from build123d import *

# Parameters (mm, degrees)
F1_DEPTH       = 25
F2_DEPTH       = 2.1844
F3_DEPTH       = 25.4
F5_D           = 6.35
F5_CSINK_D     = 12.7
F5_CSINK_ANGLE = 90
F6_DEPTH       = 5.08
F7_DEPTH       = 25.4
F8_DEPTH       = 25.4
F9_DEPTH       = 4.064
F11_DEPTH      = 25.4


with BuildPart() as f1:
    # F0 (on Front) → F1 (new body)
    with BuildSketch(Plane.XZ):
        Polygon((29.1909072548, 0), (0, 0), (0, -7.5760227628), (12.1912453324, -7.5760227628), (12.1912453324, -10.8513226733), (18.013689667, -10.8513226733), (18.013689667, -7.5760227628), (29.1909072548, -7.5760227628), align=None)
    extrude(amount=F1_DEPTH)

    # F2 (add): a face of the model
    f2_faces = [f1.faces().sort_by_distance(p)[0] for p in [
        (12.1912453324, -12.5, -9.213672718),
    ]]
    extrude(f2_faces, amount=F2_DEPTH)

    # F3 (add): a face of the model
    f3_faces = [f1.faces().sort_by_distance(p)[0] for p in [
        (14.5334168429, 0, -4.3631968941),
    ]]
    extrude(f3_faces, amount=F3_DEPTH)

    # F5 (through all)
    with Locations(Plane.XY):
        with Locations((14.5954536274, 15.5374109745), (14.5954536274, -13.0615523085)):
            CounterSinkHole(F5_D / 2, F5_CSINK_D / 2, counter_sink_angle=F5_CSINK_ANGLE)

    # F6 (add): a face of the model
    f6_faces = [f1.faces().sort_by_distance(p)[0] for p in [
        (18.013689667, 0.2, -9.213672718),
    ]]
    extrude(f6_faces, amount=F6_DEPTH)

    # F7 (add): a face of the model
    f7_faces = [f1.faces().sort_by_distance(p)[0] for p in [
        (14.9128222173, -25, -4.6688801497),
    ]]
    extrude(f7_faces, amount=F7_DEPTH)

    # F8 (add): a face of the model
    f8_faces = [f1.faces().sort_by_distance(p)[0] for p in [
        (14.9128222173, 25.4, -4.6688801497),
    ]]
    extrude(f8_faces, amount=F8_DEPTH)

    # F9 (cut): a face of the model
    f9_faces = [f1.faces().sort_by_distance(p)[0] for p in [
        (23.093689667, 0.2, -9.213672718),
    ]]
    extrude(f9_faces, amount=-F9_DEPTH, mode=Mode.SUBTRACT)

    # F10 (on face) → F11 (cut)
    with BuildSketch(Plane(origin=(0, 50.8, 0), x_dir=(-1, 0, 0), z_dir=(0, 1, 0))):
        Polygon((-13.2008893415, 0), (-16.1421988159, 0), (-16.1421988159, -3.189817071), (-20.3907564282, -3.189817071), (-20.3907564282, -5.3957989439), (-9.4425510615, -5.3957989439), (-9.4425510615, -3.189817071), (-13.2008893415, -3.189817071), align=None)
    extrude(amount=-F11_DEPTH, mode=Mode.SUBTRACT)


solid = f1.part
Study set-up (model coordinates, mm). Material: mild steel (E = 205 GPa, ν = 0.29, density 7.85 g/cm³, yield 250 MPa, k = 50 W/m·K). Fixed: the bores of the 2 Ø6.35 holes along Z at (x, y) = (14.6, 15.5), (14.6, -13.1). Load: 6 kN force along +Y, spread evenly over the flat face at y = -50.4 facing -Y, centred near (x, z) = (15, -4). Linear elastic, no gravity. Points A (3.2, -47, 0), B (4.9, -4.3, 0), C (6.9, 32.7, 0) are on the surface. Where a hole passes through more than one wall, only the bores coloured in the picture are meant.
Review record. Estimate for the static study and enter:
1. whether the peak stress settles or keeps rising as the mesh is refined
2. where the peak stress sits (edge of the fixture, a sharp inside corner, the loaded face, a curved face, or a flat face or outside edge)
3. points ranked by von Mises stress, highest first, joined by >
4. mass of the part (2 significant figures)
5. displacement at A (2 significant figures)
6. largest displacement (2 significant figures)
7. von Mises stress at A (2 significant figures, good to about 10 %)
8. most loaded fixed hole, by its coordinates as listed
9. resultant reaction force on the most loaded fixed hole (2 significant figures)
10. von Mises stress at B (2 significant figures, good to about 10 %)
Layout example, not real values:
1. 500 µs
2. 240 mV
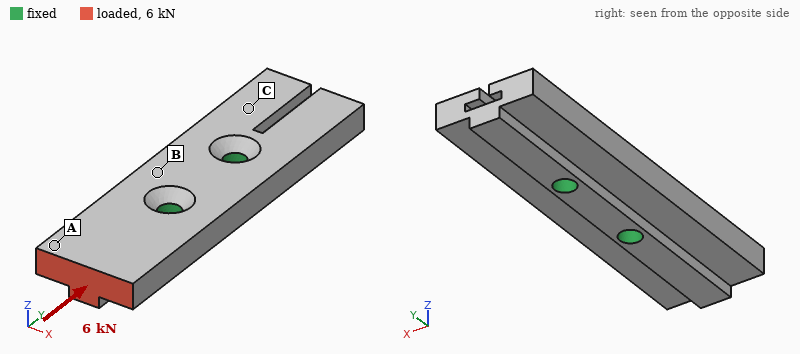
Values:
1. keeps rising
2. edge of the fixture
3. A > B > C
4. 180 g
5. 8.1 µm
6. 8.8 µm
7. 24 MPa
8. (14.6, -13.1)
9. 4.9 kN
10. 14 MPa
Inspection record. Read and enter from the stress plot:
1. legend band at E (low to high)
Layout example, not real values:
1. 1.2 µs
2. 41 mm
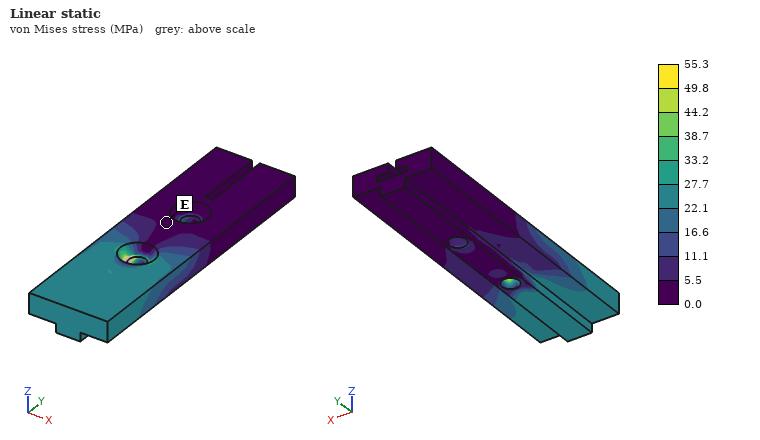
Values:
1. 0.0 to 5.5 MPa
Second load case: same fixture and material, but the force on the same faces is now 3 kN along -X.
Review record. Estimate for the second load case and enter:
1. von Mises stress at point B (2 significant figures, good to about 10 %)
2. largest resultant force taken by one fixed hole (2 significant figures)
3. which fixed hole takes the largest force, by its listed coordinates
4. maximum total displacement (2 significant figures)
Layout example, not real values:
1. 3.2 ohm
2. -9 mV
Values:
1. 37 MPa
2. 5.6 kN
3. (14.6, -13.1)
4. 43 µm
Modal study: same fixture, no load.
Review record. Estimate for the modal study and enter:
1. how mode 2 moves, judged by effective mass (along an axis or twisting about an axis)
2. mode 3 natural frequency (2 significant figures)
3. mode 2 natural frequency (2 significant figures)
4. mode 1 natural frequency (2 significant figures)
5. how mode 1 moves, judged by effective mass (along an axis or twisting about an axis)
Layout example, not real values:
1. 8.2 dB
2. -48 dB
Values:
1. along Z
2. 8100 Hz
3. 5600 Hz
4. 4900 Hz
5. along Z
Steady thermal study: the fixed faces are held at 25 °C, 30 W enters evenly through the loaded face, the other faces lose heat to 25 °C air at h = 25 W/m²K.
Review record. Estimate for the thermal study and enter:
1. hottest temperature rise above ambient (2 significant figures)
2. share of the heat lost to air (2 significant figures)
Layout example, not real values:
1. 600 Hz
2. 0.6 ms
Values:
1. 87 K
2. 12 %
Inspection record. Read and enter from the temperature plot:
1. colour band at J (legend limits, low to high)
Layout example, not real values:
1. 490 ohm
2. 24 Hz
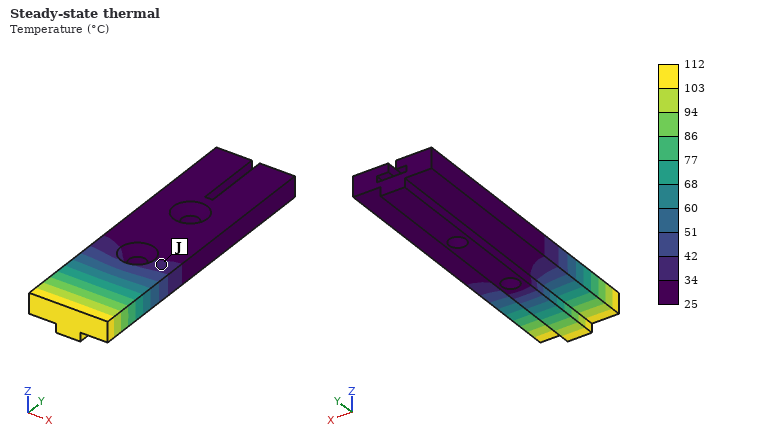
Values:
1. 34 to 42 °C
